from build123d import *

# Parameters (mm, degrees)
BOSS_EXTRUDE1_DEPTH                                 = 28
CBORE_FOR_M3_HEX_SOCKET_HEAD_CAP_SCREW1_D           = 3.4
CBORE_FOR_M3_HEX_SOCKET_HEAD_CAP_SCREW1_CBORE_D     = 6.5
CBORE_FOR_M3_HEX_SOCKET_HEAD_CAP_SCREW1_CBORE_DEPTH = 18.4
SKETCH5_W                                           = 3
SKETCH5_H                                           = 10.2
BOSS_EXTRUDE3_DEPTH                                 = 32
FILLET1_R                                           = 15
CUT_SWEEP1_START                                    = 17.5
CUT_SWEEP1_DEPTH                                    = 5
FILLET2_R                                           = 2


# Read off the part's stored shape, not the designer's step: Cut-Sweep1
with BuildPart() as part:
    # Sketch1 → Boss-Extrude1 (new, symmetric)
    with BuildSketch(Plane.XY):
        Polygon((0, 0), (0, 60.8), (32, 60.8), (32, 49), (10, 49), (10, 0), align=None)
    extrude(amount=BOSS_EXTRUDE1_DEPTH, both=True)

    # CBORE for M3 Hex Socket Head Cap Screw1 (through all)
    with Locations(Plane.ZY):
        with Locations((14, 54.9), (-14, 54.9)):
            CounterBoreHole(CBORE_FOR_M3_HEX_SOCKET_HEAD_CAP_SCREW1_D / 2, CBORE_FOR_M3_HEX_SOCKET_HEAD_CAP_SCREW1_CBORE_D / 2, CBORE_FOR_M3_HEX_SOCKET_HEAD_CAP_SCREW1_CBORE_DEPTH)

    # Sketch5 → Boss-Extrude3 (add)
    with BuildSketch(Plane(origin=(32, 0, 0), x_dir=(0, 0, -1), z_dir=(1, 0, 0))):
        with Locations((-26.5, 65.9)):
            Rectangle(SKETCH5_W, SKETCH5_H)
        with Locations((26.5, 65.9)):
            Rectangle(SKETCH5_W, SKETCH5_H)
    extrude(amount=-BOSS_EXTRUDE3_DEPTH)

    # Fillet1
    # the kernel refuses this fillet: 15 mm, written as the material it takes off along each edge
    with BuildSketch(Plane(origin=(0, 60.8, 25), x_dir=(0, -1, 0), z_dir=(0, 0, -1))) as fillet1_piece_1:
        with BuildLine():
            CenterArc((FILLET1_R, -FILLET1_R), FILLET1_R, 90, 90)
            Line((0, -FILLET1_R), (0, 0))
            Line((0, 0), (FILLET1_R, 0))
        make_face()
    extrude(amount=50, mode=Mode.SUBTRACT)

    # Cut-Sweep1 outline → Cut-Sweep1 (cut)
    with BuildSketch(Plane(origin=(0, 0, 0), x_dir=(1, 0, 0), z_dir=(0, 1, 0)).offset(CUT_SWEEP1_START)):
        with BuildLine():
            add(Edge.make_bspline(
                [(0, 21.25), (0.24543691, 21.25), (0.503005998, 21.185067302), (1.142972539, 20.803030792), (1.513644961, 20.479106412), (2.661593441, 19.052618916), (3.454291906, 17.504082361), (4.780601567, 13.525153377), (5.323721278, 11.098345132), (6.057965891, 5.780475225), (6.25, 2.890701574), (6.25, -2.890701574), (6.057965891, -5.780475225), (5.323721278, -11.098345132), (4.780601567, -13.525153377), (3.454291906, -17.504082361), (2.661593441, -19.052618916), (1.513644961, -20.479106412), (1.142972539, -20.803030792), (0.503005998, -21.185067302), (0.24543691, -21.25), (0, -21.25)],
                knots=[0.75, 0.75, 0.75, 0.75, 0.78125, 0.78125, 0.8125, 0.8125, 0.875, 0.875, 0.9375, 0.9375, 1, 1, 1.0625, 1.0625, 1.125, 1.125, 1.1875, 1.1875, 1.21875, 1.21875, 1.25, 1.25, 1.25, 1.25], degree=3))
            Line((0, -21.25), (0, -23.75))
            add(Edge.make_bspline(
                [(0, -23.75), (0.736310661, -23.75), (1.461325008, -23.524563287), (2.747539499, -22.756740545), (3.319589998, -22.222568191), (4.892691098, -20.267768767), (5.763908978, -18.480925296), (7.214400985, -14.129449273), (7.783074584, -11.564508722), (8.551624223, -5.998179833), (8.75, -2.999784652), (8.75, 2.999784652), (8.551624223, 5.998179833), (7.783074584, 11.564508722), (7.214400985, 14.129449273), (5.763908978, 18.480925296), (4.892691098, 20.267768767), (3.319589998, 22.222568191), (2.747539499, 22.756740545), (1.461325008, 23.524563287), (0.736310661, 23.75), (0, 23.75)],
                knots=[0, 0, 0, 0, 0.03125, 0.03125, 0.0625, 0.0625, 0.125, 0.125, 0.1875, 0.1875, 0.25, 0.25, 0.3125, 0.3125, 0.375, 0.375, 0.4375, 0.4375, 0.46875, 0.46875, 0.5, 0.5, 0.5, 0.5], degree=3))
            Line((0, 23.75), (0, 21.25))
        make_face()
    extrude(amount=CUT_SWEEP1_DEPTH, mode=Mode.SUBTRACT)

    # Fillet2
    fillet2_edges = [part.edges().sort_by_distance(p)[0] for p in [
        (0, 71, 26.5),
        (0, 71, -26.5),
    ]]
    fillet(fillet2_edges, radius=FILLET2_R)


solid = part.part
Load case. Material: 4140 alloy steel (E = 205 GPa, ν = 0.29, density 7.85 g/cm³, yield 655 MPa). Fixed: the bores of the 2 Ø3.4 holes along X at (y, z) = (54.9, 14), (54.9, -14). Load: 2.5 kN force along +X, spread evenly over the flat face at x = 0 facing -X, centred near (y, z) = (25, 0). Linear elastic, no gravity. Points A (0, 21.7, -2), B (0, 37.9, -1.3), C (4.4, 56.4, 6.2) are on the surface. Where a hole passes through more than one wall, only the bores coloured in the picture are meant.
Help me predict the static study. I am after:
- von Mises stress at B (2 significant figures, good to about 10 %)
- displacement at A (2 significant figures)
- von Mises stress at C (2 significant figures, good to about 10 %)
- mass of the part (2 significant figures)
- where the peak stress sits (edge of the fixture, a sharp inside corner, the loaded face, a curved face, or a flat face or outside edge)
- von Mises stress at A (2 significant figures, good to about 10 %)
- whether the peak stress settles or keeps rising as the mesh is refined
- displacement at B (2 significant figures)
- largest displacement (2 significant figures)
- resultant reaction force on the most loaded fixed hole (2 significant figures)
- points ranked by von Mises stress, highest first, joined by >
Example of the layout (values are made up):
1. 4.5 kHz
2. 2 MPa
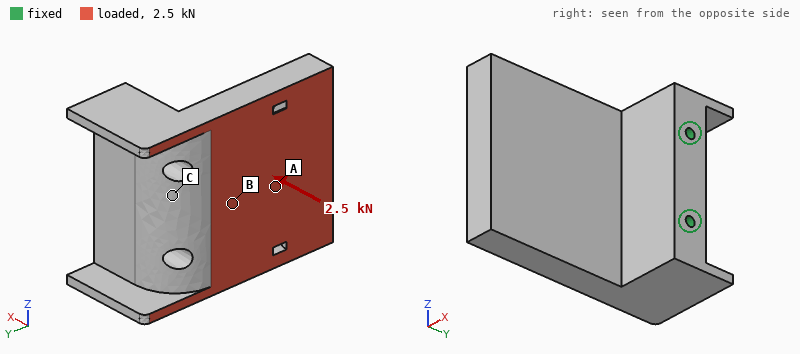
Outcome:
1. 37 MPa
2. 0.073 mm
3. 53 MPa
4. 360 g
5. edge of the fixture
6. 15 MPa
7. keeps rising
8. 0.039 mm
9. 0.13 mm
10. 1.3 kN
11. C > B > A
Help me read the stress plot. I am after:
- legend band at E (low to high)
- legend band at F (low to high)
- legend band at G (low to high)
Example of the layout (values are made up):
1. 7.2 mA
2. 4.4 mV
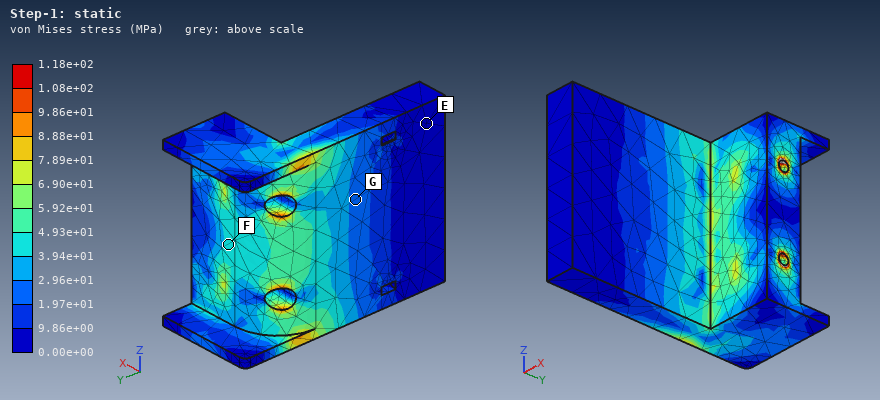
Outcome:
1. 0.00e+00 to 9.86e+00 MPa
2. 3.94e+01 to 4.93e+01 MPa
3. 1.97e+01 to 2.96e+01 MPa
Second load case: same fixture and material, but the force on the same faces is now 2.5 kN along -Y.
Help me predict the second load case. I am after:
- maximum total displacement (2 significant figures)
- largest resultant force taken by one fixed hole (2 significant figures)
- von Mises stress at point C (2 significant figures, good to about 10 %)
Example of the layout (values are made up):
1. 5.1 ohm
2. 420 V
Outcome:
1. 56 µm
2. 1.3 kN
3. 17 MPa
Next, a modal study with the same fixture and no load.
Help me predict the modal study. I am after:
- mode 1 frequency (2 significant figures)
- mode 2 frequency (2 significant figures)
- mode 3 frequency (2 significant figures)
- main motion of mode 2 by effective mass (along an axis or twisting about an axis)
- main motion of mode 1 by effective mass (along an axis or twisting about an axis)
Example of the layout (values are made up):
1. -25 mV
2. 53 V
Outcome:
1. 1900 Hz
2. 3500 Hz
3. 5700 Hz
4. along Z
5. along X
